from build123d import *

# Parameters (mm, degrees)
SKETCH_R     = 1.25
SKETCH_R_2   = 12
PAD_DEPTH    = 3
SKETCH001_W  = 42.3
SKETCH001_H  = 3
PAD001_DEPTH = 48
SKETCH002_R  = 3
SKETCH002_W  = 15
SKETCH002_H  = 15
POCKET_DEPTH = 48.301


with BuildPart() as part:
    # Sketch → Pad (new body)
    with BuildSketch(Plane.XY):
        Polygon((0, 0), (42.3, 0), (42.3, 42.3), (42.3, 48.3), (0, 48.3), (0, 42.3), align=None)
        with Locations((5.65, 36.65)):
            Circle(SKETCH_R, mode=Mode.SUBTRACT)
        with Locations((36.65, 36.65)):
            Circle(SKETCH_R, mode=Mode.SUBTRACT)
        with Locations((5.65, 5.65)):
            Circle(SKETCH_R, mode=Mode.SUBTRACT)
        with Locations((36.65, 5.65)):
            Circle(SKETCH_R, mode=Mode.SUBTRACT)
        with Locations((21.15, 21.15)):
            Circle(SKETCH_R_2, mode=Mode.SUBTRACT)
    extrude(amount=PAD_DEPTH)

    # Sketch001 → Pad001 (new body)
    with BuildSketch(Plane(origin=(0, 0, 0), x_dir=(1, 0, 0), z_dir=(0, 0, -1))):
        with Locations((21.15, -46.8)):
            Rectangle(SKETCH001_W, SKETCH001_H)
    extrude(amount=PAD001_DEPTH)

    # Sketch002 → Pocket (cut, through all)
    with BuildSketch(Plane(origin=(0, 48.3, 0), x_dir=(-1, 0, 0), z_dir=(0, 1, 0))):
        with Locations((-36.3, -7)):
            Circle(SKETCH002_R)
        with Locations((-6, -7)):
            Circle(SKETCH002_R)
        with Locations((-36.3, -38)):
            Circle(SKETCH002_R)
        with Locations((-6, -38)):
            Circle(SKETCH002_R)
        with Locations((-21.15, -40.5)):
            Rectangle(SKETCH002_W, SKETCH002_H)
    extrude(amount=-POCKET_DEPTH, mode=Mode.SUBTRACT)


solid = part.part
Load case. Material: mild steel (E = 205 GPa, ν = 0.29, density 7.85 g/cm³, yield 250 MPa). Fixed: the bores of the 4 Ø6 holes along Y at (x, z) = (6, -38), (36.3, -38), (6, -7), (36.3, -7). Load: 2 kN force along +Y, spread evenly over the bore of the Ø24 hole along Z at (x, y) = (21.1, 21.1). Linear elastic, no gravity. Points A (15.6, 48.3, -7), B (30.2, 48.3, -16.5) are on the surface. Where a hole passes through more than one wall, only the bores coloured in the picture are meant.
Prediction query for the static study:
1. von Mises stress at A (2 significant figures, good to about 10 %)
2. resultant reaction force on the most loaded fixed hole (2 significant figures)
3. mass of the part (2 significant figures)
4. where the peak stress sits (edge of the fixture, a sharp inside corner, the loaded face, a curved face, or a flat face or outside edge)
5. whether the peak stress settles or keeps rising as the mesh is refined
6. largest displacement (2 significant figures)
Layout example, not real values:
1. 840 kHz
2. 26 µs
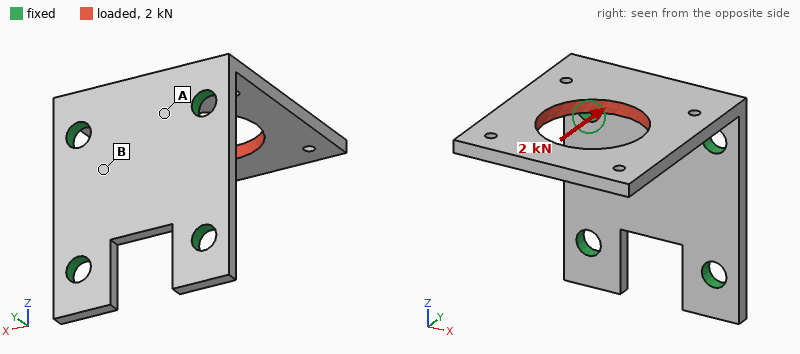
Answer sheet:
1. 51 MPa
2. 1.0 kN
3. 77 g
4. edge of the fixture
5. keeps rising
6. 0.12 mm
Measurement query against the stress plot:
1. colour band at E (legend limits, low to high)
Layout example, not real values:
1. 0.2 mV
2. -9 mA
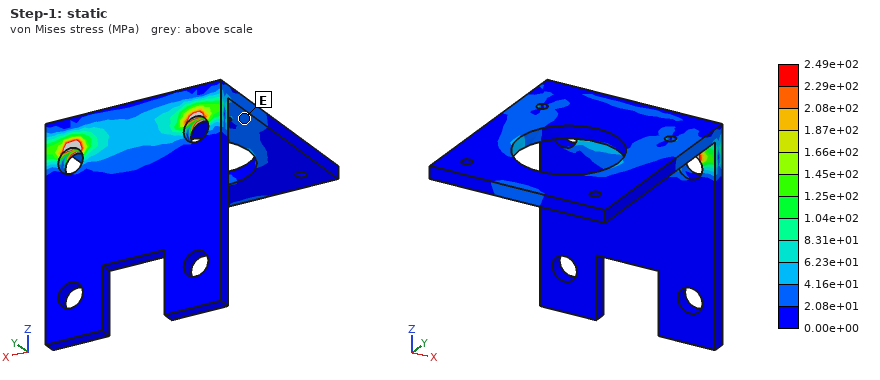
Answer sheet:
1. 2.08e+01 to 4.16e+01 MPa
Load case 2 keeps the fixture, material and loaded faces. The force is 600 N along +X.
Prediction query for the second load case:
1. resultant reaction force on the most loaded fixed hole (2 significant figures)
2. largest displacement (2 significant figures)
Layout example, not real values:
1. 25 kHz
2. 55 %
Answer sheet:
1. 580 N
2. 33 µm
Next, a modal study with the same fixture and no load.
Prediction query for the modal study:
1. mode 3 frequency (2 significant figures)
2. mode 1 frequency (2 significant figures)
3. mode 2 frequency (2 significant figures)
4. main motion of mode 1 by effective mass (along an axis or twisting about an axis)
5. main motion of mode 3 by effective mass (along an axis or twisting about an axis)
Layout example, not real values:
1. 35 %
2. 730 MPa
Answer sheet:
1. 4800 Hz
2. 930 Hz
3. 2400 Hz
4. along Z
5. along X
